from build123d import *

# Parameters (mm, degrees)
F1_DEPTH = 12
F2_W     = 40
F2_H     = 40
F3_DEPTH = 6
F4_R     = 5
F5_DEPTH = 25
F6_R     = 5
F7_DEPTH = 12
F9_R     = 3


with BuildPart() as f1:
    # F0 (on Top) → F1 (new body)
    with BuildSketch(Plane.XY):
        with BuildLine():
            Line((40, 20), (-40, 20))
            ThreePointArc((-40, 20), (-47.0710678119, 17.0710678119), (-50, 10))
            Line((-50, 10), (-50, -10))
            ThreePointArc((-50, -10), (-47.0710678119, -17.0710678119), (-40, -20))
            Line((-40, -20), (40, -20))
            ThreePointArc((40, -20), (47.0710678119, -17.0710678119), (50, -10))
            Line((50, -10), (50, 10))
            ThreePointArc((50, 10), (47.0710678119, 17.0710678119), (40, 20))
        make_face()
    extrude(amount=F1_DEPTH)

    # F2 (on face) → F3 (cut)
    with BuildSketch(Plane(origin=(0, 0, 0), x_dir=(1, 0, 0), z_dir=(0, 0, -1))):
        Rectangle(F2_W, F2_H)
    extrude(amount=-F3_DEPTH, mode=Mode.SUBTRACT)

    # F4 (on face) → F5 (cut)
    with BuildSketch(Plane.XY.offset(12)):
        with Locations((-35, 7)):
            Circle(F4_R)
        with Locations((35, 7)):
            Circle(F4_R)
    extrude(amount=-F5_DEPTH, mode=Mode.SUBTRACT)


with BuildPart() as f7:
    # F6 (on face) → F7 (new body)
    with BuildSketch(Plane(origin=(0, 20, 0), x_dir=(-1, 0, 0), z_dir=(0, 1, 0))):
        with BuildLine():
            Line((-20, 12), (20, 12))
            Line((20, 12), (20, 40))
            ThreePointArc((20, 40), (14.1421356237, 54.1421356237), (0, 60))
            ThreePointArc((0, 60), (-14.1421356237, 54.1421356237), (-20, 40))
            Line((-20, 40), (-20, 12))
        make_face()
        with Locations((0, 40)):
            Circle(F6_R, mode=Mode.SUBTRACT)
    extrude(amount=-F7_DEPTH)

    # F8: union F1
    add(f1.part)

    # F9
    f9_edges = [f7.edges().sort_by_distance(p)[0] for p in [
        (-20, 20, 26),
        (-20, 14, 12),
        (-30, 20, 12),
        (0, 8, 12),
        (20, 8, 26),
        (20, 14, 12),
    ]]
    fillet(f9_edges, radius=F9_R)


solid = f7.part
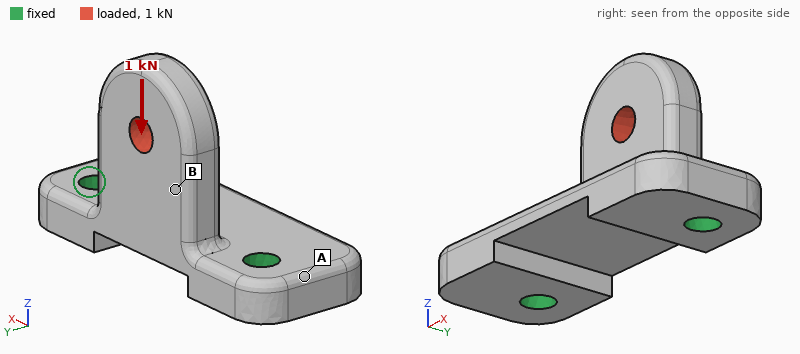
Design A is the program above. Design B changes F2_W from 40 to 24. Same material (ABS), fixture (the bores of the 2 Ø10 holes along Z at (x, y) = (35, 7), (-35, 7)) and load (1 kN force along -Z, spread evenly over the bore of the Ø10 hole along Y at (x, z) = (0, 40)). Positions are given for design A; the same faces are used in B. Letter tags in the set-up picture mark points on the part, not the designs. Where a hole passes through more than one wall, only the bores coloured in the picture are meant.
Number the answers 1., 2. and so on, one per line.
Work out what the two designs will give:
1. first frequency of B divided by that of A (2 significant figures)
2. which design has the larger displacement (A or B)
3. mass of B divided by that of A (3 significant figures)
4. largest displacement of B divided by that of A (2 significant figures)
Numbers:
1. 1.1
2. A
3. 1.07
4. 0.83
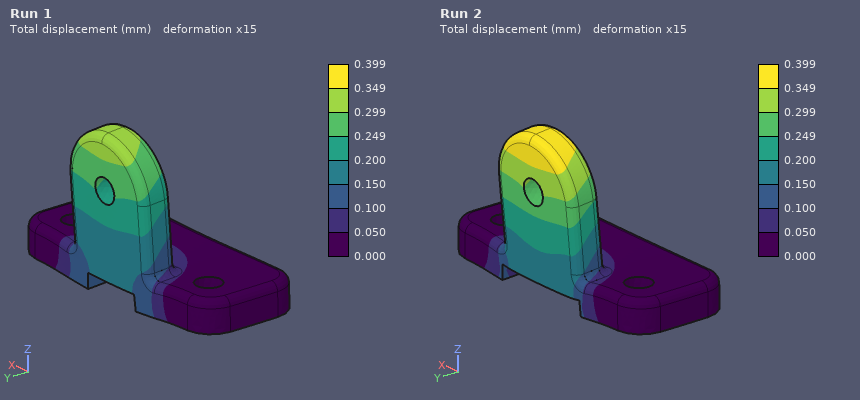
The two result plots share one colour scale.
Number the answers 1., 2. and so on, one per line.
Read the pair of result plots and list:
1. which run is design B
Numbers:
1. Run 1
